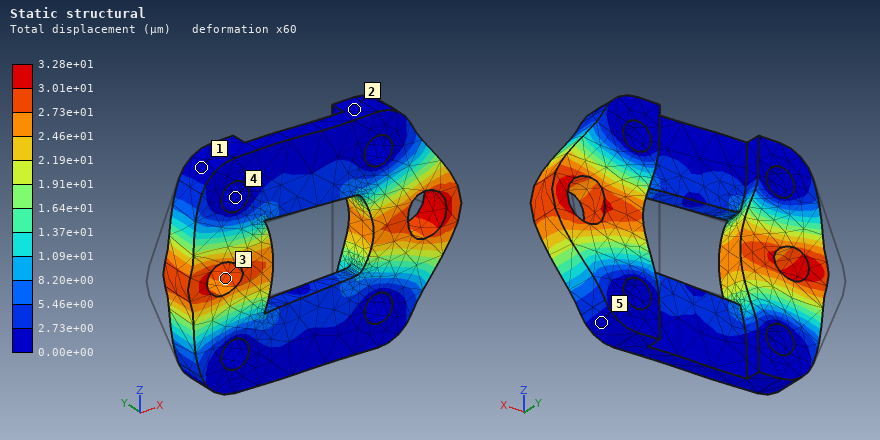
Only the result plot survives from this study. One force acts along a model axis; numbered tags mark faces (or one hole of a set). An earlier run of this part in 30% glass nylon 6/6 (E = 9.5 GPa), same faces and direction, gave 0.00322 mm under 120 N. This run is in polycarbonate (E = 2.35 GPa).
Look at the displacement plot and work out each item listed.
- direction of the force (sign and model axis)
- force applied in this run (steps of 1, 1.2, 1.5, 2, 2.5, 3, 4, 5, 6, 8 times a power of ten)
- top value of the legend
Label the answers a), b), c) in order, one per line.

a) +X
b) 300 N
c) 3.28e+01 µm
